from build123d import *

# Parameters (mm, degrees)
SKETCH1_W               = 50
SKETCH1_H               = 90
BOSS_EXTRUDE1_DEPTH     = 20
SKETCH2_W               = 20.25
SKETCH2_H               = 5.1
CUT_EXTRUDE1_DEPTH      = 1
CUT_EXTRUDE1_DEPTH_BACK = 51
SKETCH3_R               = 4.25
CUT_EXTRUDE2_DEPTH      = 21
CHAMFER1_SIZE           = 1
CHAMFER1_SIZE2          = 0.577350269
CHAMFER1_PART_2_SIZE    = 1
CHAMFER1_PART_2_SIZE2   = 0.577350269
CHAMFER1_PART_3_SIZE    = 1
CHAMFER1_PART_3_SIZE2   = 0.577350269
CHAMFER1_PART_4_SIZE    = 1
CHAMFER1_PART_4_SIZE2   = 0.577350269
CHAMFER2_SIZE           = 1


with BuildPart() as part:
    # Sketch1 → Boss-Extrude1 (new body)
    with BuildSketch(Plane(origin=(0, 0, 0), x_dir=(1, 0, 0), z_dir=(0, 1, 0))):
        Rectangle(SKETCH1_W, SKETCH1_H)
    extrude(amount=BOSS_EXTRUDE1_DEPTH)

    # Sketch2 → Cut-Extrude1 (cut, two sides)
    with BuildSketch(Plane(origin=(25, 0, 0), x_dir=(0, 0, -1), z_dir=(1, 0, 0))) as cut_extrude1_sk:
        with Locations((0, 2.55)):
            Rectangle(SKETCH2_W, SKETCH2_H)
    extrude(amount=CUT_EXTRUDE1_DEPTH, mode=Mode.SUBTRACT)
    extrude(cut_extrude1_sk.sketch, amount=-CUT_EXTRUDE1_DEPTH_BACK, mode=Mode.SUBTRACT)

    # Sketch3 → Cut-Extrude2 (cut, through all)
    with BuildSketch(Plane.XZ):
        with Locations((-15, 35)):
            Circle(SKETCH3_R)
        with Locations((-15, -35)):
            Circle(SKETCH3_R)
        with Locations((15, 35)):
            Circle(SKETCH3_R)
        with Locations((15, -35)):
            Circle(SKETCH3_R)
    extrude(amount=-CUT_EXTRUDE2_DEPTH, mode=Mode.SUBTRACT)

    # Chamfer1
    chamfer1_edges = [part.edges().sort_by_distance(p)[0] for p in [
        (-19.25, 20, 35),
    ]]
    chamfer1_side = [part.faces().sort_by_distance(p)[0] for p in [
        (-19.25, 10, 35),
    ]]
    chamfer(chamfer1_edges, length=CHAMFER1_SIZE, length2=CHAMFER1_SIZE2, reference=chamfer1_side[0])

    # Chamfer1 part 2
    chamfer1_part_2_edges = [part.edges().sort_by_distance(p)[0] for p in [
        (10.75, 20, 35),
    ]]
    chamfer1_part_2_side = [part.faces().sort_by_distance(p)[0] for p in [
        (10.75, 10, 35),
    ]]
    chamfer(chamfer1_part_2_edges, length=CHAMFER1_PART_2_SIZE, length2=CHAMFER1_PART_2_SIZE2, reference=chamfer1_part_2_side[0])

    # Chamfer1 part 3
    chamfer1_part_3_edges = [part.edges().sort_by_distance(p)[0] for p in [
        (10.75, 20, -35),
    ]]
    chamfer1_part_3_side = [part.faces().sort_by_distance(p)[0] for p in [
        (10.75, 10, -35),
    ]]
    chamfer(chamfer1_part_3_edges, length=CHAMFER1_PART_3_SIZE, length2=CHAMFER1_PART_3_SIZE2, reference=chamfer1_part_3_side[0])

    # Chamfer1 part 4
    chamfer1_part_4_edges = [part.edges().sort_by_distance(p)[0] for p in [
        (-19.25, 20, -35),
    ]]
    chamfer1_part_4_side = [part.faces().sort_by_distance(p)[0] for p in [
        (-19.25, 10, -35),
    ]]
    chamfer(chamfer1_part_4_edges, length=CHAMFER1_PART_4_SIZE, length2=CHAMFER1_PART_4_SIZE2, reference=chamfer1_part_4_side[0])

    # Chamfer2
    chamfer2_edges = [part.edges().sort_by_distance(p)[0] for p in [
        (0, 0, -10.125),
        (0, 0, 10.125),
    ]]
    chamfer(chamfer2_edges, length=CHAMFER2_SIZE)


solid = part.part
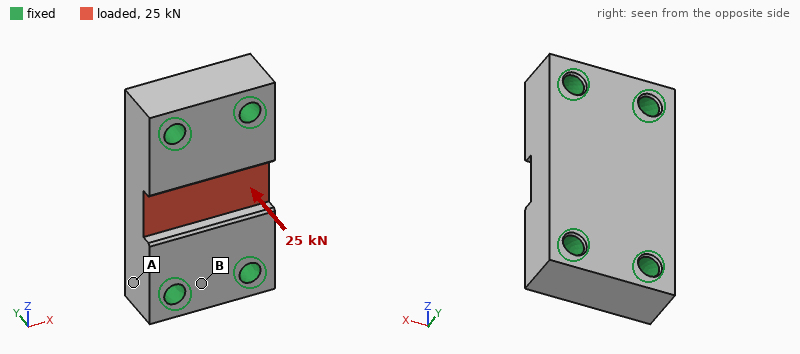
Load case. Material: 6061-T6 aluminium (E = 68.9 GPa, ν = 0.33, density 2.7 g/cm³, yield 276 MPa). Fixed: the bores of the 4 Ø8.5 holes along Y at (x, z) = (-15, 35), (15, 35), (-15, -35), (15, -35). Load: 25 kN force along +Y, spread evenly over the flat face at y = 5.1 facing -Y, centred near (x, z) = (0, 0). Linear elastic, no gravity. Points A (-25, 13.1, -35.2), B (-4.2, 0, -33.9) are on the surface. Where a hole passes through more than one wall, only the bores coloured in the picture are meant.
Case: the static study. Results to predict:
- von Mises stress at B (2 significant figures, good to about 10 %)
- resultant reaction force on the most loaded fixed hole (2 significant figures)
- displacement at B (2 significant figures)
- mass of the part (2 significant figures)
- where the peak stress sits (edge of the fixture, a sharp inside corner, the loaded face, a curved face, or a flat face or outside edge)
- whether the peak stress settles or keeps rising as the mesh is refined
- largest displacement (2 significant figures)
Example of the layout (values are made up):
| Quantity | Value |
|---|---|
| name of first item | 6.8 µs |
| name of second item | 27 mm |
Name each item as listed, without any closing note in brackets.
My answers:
| Quantity | Value |
|---|---|
| von Mises stress at B | 25 MPa |
| resultant reaction force on the most loaded fixed hole | 6.6 kN |
| displacement at B | 6.9 µm |
| mass of the part | 220 g |
| where the peak stress sits | edge of the fixture |
| whether the peak stress settles or keeps rising as the mesh is refined | keeps rising |
| largest displacement | 45 µm |
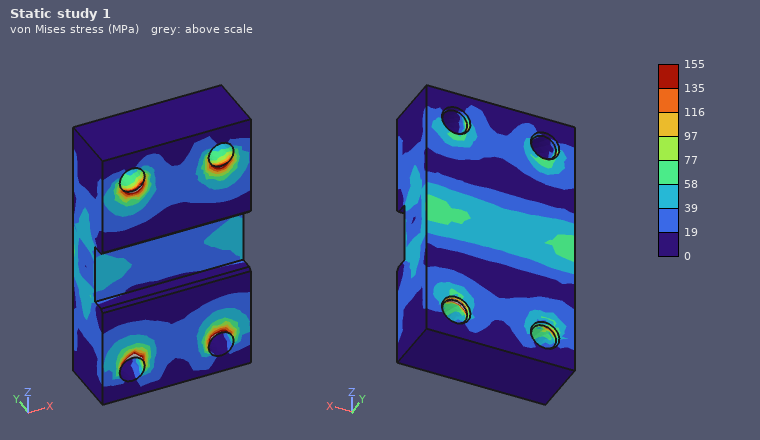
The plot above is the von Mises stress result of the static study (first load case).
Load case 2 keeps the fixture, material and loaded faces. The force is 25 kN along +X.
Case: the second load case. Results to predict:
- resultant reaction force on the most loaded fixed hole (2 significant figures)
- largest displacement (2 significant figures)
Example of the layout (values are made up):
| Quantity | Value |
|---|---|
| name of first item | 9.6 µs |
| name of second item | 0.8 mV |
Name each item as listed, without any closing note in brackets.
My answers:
| Quantity | Value |
|---|---|
| resultant reaction force on the most loaded fixed hole | 8.2 kN |
| largest displacement | 37 µm |
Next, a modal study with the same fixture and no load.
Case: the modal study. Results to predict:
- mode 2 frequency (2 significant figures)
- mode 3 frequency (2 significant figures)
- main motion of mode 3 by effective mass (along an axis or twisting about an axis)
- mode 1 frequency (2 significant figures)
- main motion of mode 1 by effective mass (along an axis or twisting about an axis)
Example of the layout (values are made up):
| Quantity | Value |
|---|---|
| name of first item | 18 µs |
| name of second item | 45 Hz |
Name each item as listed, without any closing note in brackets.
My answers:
| Quantity | Value |
|---|---|
| mode 2 frequency | 19 kHz |
| mode 3 frequency | 22 kHz |
| main motion of mode 3 by effective mass | along X |
| mode 1 frequency | 15 kHz |
| main motion of mode 1 by effective mass | along Y |
